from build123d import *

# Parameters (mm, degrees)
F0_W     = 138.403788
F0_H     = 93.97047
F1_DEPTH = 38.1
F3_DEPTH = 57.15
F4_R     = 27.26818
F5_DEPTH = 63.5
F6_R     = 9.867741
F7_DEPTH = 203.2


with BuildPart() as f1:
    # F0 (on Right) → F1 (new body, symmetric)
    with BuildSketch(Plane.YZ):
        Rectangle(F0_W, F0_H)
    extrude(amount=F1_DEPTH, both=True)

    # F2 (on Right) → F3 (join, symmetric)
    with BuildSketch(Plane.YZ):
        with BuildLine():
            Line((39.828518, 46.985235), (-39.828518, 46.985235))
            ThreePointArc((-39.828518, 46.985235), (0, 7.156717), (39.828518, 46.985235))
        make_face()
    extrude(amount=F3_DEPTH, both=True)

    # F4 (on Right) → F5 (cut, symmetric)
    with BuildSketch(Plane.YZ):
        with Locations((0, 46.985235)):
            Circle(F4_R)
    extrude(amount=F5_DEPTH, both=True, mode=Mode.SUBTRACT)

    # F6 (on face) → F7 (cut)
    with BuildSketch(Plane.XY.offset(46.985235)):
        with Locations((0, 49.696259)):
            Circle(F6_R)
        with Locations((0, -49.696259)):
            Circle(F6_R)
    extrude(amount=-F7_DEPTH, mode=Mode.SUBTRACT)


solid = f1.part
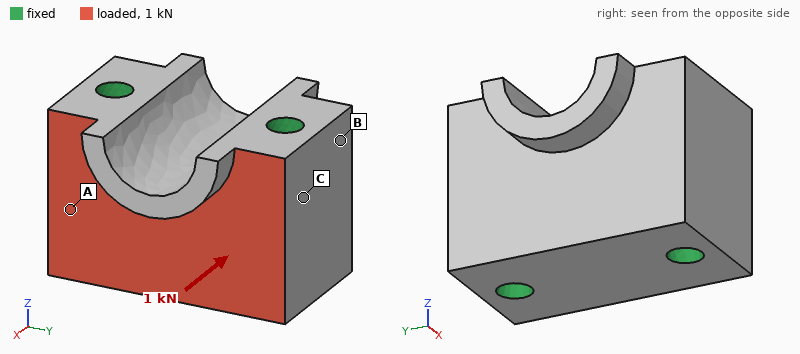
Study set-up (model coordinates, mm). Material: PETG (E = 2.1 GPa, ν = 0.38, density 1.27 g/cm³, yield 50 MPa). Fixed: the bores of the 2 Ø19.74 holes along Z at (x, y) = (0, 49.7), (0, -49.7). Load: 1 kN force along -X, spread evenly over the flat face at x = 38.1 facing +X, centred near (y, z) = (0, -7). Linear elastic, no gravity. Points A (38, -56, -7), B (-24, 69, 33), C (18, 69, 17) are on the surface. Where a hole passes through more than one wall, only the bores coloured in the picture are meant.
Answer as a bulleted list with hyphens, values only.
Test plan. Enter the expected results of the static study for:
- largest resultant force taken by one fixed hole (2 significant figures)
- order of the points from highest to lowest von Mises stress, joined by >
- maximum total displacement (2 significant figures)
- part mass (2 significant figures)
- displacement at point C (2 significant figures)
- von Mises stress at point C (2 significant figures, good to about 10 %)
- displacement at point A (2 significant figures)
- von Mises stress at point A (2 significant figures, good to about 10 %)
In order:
- 500 N
- A > C > B
- 4.2 µm
- 1.1 kg
- 0.82 µm
- 0.060 MPa
- 1.5 µm
- 0.11 MPa
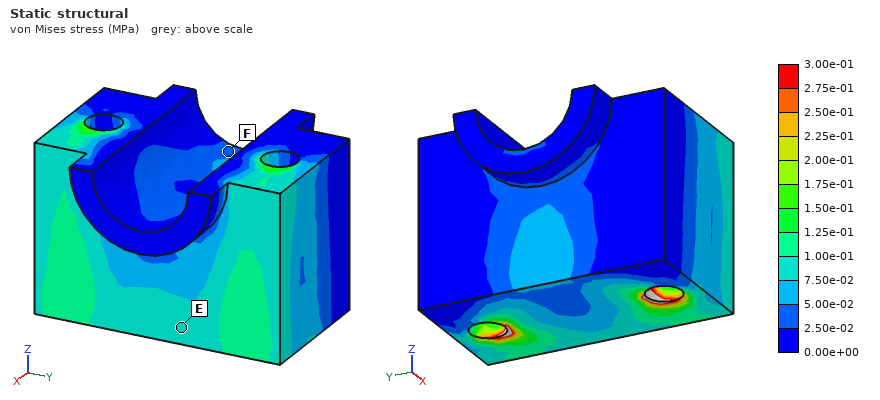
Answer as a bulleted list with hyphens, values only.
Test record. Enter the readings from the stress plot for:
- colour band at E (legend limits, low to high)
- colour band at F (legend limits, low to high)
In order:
- 7.50e-02 to 1.00e-01 MPa
- 2.50e-02 to 5.00e-02 MPa
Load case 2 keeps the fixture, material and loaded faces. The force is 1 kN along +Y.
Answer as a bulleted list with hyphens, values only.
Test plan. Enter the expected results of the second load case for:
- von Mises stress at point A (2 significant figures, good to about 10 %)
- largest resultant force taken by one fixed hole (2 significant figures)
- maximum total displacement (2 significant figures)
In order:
- 0.21 MPa
- 570 N
- 8.5 µm
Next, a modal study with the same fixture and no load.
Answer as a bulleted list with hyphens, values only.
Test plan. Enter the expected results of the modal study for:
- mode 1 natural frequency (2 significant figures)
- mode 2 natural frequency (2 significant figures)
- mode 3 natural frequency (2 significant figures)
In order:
- 3100 Hz
- 3200 Hz
- 3300 Hz
